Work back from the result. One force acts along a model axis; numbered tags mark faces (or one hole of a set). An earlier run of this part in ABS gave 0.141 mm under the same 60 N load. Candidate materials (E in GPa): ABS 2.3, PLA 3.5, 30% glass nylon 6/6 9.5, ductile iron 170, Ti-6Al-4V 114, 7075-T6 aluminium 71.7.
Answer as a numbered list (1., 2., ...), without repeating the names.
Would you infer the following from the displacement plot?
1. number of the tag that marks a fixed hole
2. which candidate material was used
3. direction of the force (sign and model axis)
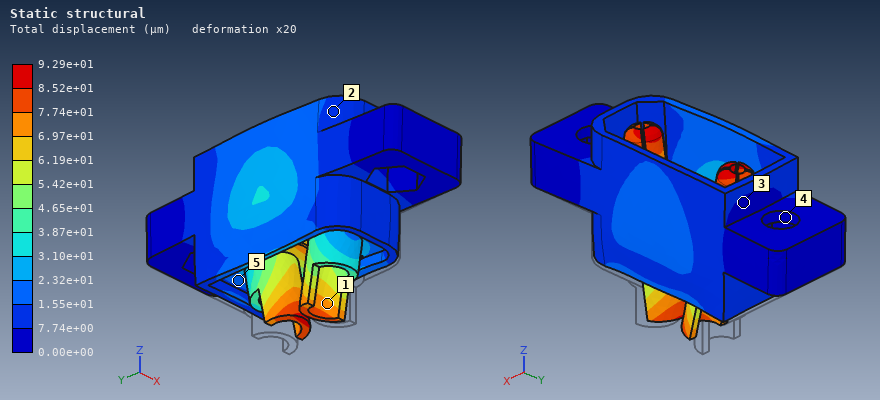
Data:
1. 4
2. PLA
3. +Z
